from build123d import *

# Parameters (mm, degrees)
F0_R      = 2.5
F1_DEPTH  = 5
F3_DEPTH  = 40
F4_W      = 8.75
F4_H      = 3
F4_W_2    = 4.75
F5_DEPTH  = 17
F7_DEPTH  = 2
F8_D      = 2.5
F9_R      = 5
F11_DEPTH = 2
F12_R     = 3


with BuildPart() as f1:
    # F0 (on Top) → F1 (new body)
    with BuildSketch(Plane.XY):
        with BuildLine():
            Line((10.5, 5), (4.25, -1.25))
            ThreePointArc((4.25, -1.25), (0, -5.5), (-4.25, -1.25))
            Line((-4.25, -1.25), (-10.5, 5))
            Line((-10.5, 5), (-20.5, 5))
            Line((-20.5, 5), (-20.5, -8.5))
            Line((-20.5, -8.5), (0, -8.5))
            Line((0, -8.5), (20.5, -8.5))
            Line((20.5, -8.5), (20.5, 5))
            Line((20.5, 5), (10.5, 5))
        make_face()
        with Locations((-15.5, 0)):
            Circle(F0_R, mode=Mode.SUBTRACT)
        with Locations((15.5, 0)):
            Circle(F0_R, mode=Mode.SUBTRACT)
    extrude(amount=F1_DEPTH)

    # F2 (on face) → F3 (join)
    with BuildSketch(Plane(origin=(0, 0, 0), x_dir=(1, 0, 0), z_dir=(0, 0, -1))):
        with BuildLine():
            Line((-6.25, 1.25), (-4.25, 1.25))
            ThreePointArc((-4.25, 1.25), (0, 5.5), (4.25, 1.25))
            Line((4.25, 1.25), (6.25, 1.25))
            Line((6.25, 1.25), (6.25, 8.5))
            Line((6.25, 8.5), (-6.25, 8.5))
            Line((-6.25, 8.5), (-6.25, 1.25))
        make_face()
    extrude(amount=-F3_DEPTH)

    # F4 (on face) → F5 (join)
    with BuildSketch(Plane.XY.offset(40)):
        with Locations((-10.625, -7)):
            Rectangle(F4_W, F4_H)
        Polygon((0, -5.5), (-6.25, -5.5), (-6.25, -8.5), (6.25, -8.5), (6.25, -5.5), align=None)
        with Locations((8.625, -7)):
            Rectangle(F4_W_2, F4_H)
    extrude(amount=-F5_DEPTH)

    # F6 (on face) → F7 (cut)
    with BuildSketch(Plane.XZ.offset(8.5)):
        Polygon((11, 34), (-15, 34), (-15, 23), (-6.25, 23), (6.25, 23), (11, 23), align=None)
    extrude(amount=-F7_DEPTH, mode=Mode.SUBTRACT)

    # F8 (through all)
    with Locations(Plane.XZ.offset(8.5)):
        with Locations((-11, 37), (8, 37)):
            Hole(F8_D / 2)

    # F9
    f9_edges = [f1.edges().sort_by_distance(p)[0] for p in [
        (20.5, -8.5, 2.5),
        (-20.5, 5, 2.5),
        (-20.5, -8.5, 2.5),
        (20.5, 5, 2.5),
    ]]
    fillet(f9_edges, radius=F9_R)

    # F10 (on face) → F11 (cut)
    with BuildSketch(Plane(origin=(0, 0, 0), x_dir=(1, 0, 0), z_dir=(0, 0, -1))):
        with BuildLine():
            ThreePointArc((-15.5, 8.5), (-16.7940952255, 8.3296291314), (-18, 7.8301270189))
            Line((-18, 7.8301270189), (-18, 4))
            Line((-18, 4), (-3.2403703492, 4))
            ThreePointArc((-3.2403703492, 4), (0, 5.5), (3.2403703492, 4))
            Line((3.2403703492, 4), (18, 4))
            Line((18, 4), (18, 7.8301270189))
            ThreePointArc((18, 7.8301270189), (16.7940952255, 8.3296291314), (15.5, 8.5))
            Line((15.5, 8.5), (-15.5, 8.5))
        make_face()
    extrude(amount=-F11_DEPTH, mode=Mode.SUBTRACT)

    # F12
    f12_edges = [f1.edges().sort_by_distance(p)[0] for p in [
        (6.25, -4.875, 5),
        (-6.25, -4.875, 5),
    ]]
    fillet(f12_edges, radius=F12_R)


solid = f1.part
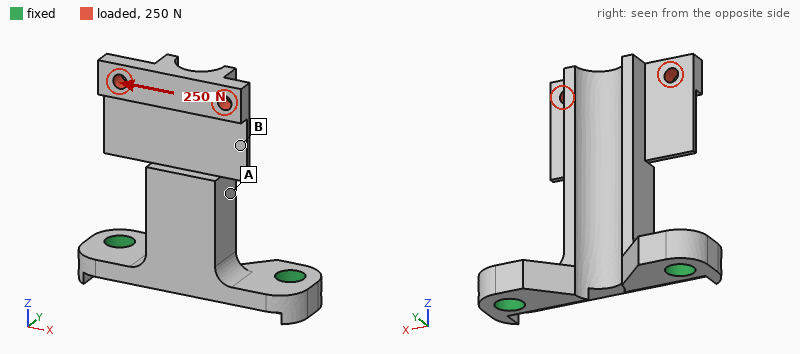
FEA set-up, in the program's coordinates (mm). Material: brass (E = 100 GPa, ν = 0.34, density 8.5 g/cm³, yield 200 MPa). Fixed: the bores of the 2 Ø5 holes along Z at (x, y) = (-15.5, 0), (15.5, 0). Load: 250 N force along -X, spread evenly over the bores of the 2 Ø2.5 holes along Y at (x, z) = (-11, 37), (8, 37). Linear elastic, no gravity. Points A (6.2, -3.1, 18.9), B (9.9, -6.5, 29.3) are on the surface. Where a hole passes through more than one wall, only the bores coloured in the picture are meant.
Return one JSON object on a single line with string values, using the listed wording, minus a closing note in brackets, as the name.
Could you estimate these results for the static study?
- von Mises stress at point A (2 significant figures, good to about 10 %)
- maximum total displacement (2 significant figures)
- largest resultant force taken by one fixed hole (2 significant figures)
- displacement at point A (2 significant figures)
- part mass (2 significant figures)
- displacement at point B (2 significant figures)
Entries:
{"von Mises stress at point A": "32 MPa", "maximum total displacement": "85 µm", "largest resultant force taken by one fixed hole": "470 N", "displacement at point A": "26 µm", "part mass": "33 g", "displacement at point B": "54 µm"}
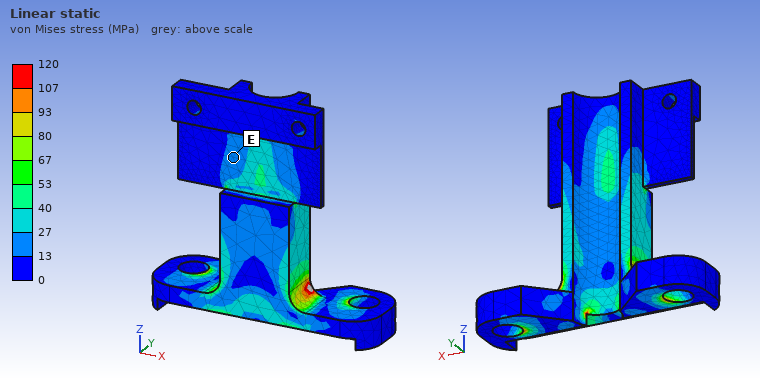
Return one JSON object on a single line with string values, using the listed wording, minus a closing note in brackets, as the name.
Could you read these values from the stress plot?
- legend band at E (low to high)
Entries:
{"legend band at E": "13 to 27 MPa"}
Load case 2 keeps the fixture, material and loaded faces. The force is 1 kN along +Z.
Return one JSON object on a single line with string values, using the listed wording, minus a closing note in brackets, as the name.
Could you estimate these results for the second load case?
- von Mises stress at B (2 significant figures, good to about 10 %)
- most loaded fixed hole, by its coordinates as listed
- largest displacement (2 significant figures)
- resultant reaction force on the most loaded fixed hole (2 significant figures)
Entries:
{"von Mises stress at B": "45 MPa", "most loaded fixed hole, by its coordinates as listed": "(-15.5, 0)", "largest displacement": "0.21 mm", "resultant reaction force on the most loaded fixed hole": "620 N"}
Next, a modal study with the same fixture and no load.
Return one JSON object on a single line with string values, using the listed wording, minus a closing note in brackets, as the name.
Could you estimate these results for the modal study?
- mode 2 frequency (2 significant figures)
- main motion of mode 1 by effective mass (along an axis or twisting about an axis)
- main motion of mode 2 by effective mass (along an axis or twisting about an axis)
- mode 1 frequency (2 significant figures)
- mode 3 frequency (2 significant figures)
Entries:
{"mode 2 frequency": "3100 Hz", "main motion of mode 1 by effective mass": "along Y", "main motion of mode 2 by effective mass": "along X", "mode 1 frequency": "1500 Hz", "mode 3 frequency": "3700 Hz"}
